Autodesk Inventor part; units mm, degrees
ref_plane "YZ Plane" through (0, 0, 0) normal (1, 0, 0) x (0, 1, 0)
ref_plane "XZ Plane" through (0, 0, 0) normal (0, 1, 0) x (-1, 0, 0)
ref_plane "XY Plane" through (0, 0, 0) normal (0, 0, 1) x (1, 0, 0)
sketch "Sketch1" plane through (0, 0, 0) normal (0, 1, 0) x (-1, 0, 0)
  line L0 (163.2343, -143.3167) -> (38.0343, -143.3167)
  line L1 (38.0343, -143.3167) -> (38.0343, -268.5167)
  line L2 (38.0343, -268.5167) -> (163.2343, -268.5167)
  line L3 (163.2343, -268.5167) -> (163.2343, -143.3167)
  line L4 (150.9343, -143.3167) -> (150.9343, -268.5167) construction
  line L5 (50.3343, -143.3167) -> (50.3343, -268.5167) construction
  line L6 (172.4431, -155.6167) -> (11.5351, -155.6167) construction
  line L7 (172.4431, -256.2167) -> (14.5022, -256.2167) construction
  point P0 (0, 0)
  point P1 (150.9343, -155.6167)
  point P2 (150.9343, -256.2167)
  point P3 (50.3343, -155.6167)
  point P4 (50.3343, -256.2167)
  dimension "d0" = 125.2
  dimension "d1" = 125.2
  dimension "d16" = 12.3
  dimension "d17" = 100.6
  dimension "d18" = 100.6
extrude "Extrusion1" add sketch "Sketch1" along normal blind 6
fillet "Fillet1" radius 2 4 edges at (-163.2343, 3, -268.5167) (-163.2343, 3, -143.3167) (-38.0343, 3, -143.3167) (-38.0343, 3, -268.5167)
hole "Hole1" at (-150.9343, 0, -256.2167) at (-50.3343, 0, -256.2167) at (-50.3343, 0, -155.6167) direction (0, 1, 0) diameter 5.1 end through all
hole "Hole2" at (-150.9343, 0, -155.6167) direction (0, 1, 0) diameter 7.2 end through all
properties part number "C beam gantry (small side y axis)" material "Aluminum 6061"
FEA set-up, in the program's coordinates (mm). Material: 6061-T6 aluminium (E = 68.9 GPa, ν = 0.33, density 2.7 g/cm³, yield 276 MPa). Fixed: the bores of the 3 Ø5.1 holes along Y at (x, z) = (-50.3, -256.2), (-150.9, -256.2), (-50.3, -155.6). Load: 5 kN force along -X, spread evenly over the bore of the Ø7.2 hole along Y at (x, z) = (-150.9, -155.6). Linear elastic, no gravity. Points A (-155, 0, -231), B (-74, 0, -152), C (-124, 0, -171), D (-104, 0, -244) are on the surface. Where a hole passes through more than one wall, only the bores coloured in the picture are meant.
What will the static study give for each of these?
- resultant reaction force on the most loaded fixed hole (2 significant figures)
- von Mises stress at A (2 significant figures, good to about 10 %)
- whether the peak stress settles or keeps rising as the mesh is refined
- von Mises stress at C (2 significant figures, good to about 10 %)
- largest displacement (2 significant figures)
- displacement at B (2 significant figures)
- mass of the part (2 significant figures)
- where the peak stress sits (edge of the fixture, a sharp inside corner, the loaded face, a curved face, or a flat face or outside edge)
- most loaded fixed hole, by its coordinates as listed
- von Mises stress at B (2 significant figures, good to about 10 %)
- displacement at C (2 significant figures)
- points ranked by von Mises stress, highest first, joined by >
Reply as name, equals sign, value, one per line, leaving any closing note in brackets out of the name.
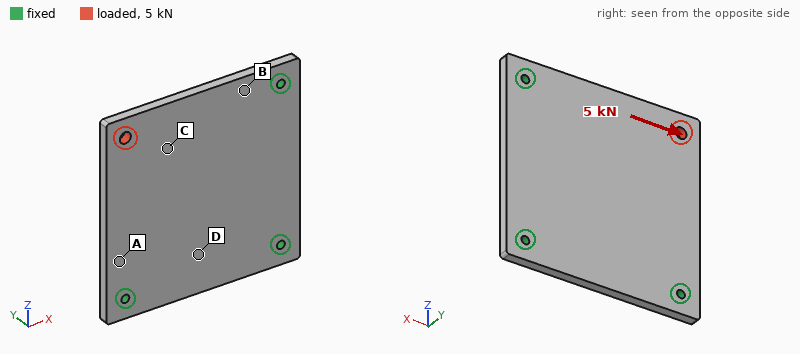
resultant reaction force on the most loaded fixed hole = 3.6 kN
von Mises stress at A = 8.6 MPa
whether the peak stress settles or keeps rising as the mesh is refined = keeps rising
von Mises stress at C = 15 MPa
largest displacement = 43 µm
displacement at B = 9.1 µm
mass of the part = 250 g
where the peak stress sits = edge of the fixture
most loaded fixed hole, by its coordinates as listed = (-50.3, -155.6)
von Mises stress at B = 22 MPa
displacement at C = 19 µm
points ranked by von Mises stress, highest first, joined by > = B > C > A > D
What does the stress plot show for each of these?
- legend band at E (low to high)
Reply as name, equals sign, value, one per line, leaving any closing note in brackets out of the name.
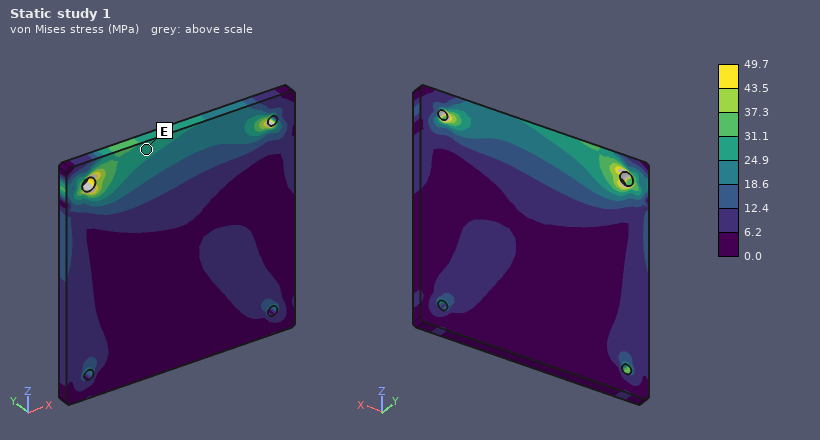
legend band at E = 24.9 to 31.1 MPa
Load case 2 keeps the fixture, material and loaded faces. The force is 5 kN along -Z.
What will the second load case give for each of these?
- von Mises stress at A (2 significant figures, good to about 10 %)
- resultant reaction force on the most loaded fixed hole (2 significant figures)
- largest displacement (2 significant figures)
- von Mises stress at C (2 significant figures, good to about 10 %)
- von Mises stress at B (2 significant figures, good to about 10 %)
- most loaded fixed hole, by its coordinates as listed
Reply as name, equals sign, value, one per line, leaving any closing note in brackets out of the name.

von Mises stress at A = 22 MPa
resultant reaction force on the most loaded fixed hole = 3.6 kN
largest displacement = 43 µm
von Mises stress at C = 7.8 MPa
von Mises stress at B = 8.7 MPa
most loaded fixed hole, by its coordinates as listed = (-150.9, -256.2)
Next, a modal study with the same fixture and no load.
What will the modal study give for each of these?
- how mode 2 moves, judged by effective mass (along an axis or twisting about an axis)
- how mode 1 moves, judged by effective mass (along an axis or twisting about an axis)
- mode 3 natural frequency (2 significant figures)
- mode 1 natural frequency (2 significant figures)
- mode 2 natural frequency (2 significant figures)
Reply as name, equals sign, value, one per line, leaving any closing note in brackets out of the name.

how mode 2 moves, judged by effective mass = along Y
how mode 1 moves, judged by effective mass = along Y
mode 3 natural frequency = 2600 Hz
mode 1 natural frequency = 720 Hz
mode 2 natural frequency = 2100 Hz
